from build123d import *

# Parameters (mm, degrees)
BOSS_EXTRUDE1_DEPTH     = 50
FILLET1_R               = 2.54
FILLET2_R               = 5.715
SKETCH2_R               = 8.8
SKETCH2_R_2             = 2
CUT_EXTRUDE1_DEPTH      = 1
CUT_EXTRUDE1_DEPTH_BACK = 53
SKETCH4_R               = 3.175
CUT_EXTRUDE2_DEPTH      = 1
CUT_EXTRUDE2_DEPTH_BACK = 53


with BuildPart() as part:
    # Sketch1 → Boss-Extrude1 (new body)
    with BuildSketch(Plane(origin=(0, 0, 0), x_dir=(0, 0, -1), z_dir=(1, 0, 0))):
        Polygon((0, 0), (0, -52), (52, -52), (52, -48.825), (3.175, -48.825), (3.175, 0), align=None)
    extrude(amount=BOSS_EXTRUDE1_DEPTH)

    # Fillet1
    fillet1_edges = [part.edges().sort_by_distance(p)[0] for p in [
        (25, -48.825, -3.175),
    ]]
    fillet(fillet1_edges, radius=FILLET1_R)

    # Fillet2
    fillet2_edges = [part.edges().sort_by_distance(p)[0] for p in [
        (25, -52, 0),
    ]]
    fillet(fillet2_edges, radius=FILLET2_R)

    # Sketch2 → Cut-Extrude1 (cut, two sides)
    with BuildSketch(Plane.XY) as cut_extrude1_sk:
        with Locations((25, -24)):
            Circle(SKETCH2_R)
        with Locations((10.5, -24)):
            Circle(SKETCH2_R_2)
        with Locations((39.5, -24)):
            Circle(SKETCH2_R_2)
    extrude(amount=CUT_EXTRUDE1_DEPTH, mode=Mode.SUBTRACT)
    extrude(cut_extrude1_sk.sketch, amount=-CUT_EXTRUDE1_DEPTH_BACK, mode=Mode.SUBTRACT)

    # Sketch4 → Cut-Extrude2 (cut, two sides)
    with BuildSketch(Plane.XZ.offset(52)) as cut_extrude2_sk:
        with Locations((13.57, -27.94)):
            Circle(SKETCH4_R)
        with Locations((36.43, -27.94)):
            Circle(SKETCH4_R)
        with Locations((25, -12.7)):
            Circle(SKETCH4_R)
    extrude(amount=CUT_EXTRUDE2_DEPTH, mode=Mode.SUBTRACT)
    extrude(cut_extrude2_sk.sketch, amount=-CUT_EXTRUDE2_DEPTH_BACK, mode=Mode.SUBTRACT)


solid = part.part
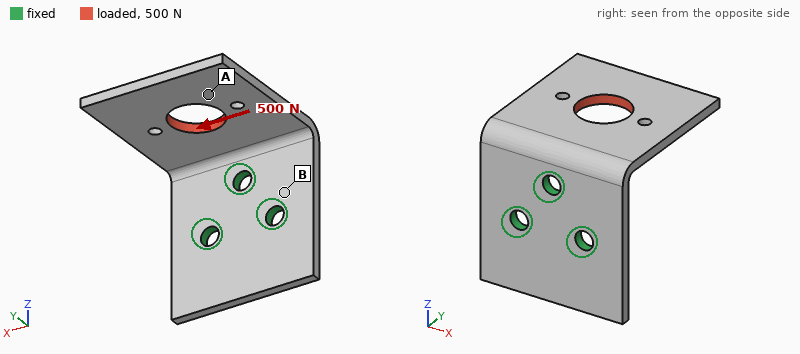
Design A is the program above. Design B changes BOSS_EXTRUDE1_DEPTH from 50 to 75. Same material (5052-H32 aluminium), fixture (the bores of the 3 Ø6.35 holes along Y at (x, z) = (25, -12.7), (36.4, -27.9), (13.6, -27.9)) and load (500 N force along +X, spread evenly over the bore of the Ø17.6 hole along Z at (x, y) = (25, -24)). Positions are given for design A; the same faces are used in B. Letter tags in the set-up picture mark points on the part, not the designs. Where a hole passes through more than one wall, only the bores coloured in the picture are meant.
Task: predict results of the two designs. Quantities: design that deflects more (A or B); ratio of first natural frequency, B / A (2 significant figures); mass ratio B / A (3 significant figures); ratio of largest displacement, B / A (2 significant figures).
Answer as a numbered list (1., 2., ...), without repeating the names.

1. B
2. 0.92
3. 1.54
4. 1.1
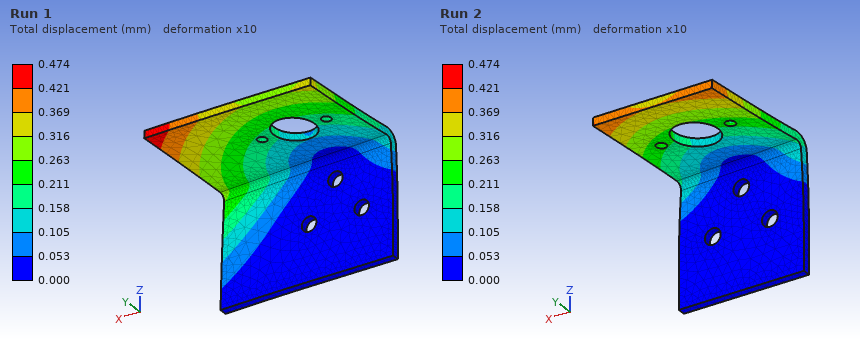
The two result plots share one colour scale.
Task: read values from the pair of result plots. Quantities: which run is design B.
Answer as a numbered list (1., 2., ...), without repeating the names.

1. Run 1
